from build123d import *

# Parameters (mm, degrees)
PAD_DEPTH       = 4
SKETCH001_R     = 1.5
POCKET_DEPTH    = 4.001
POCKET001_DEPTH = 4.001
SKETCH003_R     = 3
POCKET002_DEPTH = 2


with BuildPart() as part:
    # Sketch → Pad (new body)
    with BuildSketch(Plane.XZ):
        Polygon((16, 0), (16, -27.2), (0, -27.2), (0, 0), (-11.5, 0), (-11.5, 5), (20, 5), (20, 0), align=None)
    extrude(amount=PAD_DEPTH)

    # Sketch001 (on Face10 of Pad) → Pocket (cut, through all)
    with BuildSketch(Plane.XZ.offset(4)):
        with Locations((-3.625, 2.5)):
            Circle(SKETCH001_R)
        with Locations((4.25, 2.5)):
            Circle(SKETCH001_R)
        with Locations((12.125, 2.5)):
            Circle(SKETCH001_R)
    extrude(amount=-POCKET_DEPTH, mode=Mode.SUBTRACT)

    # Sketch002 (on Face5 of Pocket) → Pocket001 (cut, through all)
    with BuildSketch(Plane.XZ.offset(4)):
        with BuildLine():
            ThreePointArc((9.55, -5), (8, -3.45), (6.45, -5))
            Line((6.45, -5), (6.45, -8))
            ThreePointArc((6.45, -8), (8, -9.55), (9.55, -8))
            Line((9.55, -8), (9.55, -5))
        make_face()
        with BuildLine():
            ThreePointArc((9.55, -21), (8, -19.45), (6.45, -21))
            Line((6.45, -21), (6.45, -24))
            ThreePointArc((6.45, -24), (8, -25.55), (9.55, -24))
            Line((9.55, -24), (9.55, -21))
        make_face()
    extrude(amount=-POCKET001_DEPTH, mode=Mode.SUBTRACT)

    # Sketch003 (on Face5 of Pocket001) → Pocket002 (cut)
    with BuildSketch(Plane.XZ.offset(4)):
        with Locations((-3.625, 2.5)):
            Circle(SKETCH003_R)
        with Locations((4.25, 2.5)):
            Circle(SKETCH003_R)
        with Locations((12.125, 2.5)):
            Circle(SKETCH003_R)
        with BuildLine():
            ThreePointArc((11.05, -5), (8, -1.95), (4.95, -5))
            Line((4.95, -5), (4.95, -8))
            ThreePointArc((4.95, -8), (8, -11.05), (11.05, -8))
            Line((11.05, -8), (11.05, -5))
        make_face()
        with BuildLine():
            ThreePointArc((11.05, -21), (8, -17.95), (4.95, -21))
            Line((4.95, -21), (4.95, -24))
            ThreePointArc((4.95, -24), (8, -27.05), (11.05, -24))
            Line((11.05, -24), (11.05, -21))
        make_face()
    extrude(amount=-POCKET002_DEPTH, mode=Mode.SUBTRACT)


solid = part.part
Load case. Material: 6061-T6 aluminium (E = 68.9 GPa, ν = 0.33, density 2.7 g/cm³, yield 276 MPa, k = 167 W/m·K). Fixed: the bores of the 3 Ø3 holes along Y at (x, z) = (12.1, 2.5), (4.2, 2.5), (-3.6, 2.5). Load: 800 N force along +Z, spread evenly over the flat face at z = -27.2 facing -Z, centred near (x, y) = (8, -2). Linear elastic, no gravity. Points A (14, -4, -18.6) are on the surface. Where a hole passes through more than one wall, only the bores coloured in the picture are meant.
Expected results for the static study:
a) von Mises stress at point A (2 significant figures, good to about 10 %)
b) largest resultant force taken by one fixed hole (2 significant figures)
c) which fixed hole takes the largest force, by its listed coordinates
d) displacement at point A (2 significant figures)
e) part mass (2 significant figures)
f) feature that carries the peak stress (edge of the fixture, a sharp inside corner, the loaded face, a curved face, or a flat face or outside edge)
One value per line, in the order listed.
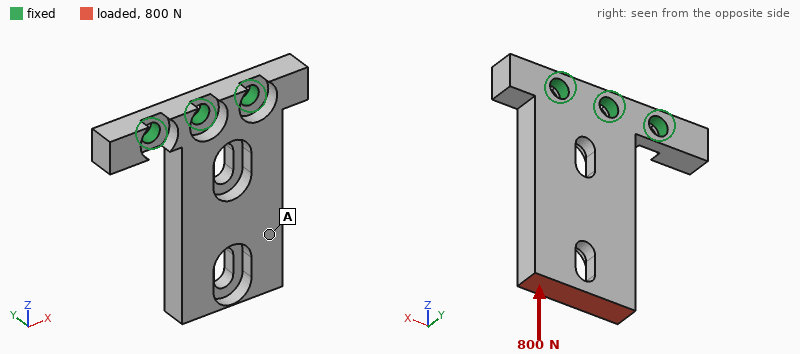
21 MPa
410 N
(12.1, 2.5)
28 µm
5.2 g
the loaded face
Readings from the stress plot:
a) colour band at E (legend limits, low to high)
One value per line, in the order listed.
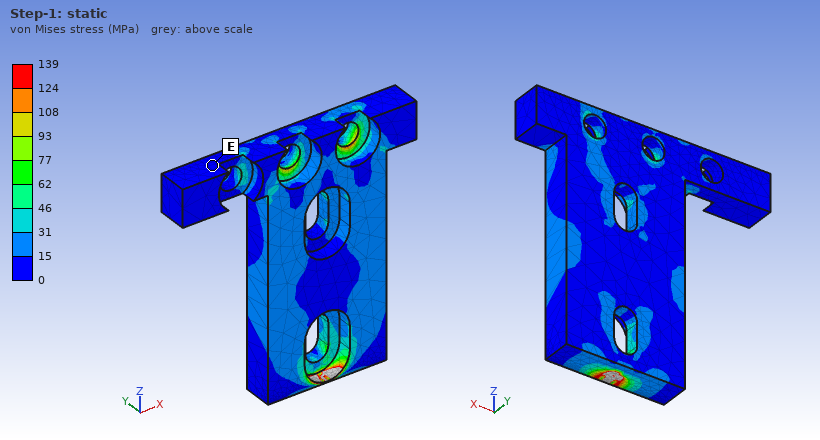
0 to 15 MPa
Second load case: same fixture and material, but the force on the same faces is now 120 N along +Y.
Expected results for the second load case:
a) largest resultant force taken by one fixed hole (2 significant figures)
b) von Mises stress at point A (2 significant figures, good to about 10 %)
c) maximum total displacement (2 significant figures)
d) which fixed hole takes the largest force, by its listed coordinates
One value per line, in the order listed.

160 N
32 MPa
0.32 mm
(4.2, 2.5)
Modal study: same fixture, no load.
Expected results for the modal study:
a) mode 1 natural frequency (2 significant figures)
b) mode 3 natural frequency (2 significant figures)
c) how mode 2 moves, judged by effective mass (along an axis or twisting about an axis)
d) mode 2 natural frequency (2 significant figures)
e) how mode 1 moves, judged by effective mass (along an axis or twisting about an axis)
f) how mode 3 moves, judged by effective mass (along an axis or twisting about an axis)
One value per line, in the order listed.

3000 Hz
11 kHz
along X
10 kHz
along Y
along X
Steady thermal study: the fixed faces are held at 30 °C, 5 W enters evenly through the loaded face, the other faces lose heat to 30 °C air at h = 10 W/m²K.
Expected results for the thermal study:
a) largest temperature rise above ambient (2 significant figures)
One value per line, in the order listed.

20 K
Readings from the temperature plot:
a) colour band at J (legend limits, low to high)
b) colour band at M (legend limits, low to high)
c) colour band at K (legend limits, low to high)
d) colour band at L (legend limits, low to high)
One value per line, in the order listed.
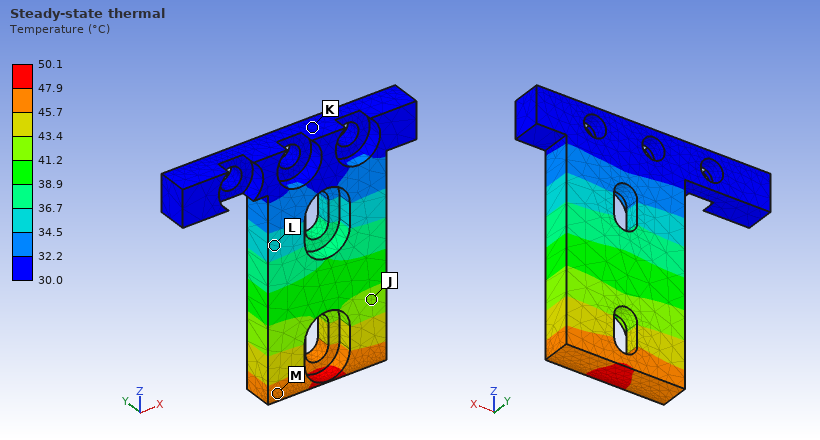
41.2 to 43.4 °C
45.7 to 47.9 °C
30.0 to 32.2 °C
34.5 to 36.7 °C
